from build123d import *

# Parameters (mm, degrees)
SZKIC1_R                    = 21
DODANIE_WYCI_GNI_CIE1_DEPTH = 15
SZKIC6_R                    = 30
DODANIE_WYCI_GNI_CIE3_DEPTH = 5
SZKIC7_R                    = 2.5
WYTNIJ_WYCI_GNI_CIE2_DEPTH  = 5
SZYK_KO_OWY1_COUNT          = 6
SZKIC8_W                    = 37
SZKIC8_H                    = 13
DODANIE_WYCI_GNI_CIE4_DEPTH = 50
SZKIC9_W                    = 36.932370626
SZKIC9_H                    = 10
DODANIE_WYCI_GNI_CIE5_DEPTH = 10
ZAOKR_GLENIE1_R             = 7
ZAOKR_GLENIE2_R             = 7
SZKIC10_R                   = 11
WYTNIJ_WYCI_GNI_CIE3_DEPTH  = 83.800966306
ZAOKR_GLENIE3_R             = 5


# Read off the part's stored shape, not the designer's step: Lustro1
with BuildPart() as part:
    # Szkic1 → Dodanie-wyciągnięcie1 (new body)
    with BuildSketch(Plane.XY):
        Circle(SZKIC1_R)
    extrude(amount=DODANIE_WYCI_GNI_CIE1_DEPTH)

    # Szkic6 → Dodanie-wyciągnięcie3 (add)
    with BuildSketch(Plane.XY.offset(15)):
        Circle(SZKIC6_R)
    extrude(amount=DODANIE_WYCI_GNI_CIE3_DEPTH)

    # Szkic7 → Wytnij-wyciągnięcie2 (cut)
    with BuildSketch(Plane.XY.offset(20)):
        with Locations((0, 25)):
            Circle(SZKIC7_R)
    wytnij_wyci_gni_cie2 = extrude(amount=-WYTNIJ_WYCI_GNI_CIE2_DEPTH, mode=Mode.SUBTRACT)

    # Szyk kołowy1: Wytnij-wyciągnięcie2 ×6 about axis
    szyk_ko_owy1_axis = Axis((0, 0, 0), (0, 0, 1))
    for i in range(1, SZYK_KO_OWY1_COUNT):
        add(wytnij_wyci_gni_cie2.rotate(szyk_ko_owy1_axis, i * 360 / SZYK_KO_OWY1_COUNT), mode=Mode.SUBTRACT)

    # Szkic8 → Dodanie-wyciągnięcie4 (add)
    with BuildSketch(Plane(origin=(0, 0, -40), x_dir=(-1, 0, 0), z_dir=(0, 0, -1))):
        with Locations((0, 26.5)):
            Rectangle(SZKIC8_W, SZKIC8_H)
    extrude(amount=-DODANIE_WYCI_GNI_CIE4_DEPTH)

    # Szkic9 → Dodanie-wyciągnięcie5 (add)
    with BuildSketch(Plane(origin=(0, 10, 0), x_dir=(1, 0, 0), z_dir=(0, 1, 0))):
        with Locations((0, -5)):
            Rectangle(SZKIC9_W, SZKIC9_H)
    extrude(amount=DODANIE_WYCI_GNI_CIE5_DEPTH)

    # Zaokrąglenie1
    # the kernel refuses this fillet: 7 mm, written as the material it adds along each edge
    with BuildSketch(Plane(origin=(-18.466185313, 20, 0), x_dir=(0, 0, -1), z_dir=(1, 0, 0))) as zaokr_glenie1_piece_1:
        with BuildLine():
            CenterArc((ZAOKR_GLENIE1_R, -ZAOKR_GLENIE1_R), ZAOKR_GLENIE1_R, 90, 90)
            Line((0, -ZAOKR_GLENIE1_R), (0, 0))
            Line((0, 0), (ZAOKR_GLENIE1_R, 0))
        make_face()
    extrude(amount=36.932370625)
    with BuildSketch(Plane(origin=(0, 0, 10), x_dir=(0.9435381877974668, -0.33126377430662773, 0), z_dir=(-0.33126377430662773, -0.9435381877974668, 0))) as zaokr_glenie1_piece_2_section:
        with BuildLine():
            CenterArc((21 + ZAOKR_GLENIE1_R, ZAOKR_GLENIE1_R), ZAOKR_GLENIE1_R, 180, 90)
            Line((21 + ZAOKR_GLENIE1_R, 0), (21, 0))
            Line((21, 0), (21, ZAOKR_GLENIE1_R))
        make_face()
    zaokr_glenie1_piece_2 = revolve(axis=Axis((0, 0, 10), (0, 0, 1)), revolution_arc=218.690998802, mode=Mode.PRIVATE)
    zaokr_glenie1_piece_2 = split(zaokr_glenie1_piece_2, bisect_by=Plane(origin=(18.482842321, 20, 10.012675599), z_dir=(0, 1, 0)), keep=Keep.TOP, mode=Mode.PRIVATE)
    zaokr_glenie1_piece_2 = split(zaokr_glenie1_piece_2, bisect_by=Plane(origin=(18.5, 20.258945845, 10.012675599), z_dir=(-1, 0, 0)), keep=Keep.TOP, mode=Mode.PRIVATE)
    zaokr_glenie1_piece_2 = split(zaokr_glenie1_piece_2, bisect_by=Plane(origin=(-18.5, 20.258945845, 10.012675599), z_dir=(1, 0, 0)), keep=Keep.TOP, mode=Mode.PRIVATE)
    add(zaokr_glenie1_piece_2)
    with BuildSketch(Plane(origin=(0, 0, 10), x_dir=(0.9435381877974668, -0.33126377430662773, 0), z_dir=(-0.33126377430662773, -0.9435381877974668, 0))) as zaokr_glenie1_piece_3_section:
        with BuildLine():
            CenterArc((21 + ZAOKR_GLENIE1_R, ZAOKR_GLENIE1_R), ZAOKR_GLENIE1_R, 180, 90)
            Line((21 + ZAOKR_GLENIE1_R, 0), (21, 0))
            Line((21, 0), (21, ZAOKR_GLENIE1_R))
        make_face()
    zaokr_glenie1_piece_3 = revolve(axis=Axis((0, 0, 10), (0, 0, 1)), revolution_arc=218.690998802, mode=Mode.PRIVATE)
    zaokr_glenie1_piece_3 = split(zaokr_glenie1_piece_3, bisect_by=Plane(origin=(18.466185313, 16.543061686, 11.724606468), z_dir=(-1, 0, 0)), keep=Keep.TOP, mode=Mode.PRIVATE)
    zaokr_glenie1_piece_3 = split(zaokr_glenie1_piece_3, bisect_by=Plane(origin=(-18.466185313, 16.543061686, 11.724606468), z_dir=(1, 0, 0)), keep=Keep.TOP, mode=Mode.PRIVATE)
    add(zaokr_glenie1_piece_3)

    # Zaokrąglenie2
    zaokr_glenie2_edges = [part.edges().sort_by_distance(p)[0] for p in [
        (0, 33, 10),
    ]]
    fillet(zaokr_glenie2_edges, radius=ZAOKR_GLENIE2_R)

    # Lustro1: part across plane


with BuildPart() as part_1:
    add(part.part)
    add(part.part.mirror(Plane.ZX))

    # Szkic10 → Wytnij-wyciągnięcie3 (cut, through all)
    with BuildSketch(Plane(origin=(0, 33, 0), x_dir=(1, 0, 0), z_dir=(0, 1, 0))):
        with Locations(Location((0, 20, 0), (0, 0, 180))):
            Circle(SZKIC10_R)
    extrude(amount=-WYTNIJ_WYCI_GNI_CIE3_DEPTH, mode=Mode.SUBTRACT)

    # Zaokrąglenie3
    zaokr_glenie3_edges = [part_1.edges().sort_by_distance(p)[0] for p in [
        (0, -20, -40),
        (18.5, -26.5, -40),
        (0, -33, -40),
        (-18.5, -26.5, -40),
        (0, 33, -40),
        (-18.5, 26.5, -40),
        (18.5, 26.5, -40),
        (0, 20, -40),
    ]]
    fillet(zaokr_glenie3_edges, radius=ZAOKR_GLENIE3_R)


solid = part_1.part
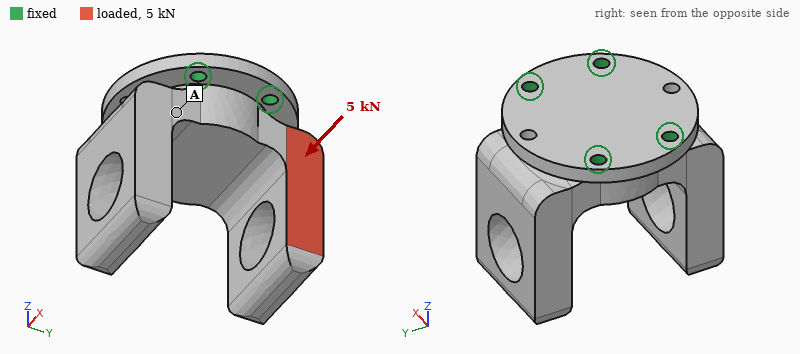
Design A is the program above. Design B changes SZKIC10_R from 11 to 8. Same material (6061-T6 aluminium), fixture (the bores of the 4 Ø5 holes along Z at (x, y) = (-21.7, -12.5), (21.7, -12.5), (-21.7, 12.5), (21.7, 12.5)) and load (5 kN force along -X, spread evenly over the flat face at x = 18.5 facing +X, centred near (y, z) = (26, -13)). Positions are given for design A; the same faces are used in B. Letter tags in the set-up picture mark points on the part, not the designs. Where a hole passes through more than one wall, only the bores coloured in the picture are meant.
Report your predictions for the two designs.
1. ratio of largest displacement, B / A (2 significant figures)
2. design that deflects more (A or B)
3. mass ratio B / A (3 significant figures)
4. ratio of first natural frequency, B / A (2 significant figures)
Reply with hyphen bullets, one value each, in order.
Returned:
- 0.87
- A
- 1.06
- 0.96
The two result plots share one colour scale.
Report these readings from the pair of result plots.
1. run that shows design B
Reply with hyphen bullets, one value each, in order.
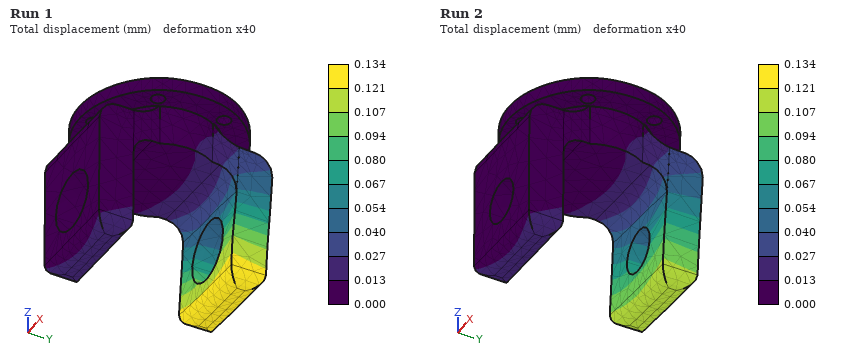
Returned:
- Run 2
